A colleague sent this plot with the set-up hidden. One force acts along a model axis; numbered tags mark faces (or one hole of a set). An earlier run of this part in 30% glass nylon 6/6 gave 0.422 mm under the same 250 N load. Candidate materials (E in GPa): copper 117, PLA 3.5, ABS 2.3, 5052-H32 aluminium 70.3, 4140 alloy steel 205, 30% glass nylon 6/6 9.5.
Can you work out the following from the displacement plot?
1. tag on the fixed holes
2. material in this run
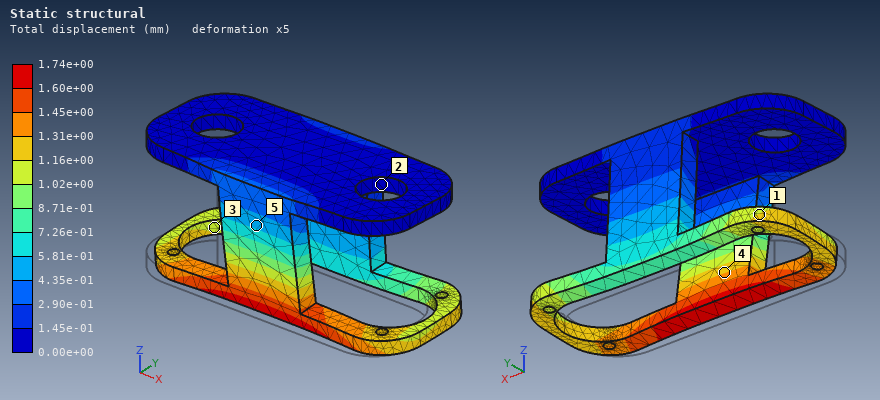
2
ABS
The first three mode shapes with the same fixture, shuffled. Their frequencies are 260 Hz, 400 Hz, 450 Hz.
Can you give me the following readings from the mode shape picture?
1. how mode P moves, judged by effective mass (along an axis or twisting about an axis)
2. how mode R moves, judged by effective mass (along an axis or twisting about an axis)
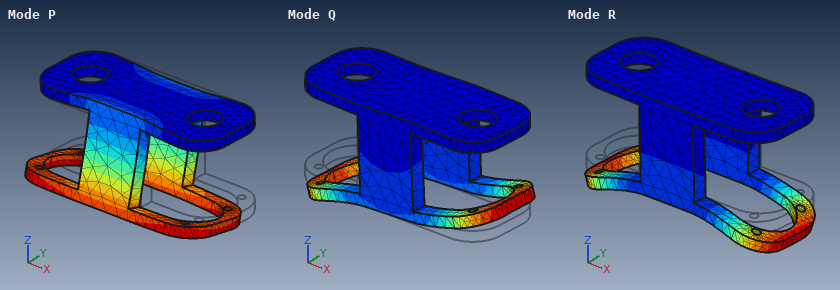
along Y
along Z
